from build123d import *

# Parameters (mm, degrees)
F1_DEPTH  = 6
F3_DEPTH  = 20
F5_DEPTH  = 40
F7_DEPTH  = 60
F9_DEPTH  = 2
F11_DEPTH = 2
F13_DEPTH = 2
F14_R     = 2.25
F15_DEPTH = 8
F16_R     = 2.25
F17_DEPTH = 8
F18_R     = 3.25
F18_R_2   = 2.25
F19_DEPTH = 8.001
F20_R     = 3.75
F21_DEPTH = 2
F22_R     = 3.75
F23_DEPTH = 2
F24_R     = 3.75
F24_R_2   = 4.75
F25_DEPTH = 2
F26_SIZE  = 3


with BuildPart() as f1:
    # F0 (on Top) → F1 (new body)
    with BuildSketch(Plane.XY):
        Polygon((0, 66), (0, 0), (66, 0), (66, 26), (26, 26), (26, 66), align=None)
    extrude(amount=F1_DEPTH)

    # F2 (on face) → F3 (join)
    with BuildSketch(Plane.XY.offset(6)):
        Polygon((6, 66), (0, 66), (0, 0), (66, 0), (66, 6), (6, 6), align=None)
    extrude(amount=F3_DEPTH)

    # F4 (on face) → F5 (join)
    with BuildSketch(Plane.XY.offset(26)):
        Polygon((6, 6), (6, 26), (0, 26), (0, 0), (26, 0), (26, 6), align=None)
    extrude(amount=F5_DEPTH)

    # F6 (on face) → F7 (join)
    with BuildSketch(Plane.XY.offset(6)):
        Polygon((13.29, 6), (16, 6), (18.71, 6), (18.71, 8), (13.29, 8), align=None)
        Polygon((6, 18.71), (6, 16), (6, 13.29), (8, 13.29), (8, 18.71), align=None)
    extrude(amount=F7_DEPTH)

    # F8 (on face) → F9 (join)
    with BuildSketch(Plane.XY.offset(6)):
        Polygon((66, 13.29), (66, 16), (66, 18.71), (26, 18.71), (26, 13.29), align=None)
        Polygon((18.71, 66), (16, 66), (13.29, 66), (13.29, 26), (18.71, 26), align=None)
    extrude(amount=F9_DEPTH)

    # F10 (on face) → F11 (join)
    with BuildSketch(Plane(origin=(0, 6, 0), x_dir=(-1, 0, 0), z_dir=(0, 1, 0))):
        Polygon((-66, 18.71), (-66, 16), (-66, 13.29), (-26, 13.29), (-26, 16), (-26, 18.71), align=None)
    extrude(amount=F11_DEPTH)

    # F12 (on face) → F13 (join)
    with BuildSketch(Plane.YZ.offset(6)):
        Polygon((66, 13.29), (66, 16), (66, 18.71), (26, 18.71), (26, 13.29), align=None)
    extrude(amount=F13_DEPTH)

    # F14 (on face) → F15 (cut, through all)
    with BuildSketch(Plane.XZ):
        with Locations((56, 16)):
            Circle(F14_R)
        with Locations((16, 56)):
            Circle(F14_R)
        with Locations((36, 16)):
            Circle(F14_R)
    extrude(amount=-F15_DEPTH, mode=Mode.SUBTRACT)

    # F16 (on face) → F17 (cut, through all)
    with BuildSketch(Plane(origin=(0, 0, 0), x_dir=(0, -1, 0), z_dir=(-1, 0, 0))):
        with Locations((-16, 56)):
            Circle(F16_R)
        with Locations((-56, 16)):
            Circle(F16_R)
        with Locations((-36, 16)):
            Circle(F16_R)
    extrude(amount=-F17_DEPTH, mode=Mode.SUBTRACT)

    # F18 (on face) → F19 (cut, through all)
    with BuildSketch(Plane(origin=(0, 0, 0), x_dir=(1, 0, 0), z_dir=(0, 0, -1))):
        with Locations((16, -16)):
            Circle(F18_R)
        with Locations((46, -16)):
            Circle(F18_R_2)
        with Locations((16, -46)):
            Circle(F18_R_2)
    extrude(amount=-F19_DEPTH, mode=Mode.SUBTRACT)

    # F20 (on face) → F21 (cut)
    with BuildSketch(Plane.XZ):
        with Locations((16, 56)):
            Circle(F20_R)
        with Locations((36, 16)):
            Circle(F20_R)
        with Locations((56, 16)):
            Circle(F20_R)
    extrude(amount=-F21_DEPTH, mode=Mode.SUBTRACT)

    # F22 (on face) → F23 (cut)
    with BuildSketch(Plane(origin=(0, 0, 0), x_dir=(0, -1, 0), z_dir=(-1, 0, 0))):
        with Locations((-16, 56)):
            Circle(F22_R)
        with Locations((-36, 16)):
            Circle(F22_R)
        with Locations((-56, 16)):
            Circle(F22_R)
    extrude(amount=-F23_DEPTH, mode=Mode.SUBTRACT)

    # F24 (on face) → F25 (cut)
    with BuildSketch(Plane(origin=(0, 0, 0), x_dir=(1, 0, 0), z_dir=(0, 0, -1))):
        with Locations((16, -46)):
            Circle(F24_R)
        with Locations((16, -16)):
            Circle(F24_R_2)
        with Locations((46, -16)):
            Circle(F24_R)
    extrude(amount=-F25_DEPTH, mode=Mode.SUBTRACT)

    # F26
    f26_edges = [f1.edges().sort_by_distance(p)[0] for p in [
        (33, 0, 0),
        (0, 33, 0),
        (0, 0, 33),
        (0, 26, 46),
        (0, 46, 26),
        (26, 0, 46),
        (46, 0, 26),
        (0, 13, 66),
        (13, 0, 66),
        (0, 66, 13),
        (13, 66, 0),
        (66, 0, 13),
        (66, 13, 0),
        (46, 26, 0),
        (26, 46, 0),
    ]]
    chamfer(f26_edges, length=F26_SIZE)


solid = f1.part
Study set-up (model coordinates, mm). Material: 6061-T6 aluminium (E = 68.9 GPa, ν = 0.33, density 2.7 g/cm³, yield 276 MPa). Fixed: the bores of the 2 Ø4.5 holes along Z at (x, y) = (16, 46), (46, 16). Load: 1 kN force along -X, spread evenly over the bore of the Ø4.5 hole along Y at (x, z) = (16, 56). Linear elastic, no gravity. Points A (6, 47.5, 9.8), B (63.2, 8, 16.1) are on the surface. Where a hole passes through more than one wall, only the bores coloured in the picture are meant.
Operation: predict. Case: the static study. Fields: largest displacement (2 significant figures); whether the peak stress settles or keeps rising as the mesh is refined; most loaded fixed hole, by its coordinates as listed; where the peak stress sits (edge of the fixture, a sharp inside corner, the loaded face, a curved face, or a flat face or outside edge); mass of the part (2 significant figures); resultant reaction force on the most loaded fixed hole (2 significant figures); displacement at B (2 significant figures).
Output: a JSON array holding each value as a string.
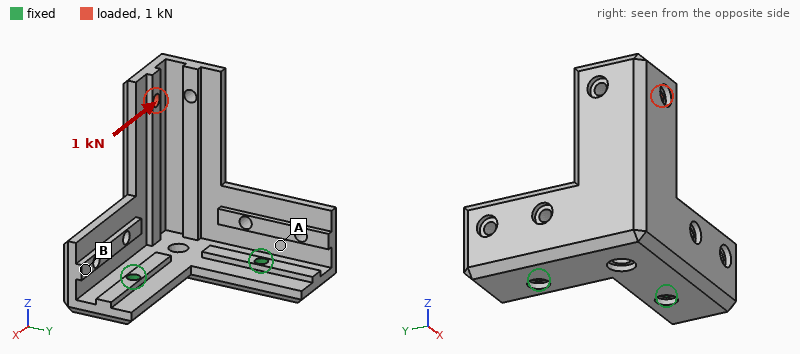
["0.58 mm", "keeps rising", "(46, 16)", "edge of the fixture", "110 g", "1.2 kN", "0.11 mm"]
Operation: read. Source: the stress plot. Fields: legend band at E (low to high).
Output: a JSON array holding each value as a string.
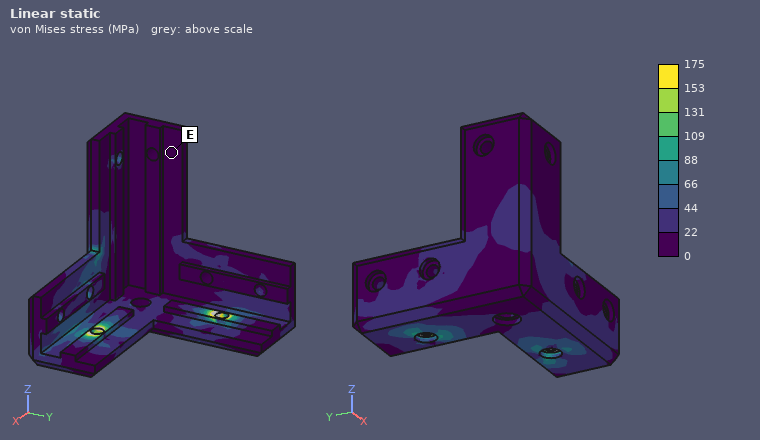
["0 to 22 MPa"]
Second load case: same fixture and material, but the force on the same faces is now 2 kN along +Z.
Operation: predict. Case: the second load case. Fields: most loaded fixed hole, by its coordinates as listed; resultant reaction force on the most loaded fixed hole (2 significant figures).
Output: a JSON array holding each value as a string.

["(46, 16)", "1.3 kN"]
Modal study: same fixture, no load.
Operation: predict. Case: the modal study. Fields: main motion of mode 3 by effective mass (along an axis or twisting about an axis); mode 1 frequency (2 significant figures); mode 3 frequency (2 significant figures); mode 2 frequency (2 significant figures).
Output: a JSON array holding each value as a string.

["along Z", "1100 Hz", "4500 Hz", "2700 Hz"]
